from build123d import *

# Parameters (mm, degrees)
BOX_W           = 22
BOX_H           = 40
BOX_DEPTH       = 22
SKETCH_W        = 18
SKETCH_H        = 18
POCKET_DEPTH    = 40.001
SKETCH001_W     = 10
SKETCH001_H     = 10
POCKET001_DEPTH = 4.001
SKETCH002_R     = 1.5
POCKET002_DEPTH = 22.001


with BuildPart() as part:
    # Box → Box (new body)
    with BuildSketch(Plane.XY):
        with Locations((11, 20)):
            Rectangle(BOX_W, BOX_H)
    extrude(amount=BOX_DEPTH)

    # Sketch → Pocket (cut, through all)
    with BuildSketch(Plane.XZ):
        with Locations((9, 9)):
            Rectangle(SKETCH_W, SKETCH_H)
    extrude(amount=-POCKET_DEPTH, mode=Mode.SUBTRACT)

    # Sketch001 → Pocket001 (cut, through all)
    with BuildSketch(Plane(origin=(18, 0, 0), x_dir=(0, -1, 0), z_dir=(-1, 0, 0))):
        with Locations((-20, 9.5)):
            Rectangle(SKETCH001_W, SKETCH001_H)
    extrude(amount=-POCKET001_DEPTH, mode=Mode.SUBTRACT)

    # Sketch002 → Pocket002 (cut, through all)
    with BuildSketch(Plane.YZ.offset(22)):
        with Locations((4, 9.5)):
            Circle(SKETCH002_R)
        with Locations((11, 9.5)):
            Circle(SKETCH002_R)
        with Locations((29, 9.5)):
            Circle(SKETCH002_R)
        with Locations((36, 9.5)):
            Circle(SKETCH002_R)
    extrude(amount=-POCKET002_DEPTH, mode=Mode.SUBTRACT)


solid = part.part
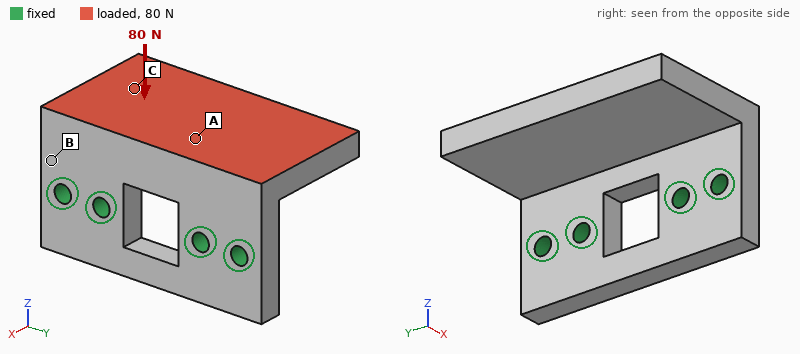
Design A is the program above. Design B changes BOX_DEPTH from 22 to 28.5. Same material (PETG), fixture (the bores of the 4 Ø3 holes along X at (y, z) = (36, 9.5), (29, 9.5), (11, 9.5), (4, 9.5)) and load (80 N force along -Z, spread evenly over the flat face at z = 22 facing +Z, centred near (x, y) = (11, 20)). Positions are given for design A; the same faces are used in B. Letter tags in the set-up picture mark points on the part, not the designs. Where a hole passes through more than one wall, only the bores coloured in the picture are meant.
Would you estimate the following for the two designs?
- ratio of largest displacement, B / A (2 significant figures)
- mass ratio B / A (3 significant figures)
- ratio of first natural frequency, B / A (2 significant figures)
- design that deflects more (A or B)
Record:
0.89
1.97
0.58
A
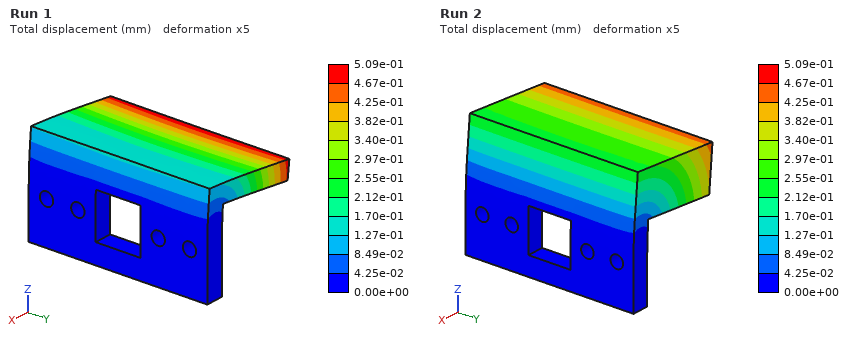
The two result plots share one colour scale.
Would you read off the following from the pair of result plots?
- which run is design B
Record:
Run 2
